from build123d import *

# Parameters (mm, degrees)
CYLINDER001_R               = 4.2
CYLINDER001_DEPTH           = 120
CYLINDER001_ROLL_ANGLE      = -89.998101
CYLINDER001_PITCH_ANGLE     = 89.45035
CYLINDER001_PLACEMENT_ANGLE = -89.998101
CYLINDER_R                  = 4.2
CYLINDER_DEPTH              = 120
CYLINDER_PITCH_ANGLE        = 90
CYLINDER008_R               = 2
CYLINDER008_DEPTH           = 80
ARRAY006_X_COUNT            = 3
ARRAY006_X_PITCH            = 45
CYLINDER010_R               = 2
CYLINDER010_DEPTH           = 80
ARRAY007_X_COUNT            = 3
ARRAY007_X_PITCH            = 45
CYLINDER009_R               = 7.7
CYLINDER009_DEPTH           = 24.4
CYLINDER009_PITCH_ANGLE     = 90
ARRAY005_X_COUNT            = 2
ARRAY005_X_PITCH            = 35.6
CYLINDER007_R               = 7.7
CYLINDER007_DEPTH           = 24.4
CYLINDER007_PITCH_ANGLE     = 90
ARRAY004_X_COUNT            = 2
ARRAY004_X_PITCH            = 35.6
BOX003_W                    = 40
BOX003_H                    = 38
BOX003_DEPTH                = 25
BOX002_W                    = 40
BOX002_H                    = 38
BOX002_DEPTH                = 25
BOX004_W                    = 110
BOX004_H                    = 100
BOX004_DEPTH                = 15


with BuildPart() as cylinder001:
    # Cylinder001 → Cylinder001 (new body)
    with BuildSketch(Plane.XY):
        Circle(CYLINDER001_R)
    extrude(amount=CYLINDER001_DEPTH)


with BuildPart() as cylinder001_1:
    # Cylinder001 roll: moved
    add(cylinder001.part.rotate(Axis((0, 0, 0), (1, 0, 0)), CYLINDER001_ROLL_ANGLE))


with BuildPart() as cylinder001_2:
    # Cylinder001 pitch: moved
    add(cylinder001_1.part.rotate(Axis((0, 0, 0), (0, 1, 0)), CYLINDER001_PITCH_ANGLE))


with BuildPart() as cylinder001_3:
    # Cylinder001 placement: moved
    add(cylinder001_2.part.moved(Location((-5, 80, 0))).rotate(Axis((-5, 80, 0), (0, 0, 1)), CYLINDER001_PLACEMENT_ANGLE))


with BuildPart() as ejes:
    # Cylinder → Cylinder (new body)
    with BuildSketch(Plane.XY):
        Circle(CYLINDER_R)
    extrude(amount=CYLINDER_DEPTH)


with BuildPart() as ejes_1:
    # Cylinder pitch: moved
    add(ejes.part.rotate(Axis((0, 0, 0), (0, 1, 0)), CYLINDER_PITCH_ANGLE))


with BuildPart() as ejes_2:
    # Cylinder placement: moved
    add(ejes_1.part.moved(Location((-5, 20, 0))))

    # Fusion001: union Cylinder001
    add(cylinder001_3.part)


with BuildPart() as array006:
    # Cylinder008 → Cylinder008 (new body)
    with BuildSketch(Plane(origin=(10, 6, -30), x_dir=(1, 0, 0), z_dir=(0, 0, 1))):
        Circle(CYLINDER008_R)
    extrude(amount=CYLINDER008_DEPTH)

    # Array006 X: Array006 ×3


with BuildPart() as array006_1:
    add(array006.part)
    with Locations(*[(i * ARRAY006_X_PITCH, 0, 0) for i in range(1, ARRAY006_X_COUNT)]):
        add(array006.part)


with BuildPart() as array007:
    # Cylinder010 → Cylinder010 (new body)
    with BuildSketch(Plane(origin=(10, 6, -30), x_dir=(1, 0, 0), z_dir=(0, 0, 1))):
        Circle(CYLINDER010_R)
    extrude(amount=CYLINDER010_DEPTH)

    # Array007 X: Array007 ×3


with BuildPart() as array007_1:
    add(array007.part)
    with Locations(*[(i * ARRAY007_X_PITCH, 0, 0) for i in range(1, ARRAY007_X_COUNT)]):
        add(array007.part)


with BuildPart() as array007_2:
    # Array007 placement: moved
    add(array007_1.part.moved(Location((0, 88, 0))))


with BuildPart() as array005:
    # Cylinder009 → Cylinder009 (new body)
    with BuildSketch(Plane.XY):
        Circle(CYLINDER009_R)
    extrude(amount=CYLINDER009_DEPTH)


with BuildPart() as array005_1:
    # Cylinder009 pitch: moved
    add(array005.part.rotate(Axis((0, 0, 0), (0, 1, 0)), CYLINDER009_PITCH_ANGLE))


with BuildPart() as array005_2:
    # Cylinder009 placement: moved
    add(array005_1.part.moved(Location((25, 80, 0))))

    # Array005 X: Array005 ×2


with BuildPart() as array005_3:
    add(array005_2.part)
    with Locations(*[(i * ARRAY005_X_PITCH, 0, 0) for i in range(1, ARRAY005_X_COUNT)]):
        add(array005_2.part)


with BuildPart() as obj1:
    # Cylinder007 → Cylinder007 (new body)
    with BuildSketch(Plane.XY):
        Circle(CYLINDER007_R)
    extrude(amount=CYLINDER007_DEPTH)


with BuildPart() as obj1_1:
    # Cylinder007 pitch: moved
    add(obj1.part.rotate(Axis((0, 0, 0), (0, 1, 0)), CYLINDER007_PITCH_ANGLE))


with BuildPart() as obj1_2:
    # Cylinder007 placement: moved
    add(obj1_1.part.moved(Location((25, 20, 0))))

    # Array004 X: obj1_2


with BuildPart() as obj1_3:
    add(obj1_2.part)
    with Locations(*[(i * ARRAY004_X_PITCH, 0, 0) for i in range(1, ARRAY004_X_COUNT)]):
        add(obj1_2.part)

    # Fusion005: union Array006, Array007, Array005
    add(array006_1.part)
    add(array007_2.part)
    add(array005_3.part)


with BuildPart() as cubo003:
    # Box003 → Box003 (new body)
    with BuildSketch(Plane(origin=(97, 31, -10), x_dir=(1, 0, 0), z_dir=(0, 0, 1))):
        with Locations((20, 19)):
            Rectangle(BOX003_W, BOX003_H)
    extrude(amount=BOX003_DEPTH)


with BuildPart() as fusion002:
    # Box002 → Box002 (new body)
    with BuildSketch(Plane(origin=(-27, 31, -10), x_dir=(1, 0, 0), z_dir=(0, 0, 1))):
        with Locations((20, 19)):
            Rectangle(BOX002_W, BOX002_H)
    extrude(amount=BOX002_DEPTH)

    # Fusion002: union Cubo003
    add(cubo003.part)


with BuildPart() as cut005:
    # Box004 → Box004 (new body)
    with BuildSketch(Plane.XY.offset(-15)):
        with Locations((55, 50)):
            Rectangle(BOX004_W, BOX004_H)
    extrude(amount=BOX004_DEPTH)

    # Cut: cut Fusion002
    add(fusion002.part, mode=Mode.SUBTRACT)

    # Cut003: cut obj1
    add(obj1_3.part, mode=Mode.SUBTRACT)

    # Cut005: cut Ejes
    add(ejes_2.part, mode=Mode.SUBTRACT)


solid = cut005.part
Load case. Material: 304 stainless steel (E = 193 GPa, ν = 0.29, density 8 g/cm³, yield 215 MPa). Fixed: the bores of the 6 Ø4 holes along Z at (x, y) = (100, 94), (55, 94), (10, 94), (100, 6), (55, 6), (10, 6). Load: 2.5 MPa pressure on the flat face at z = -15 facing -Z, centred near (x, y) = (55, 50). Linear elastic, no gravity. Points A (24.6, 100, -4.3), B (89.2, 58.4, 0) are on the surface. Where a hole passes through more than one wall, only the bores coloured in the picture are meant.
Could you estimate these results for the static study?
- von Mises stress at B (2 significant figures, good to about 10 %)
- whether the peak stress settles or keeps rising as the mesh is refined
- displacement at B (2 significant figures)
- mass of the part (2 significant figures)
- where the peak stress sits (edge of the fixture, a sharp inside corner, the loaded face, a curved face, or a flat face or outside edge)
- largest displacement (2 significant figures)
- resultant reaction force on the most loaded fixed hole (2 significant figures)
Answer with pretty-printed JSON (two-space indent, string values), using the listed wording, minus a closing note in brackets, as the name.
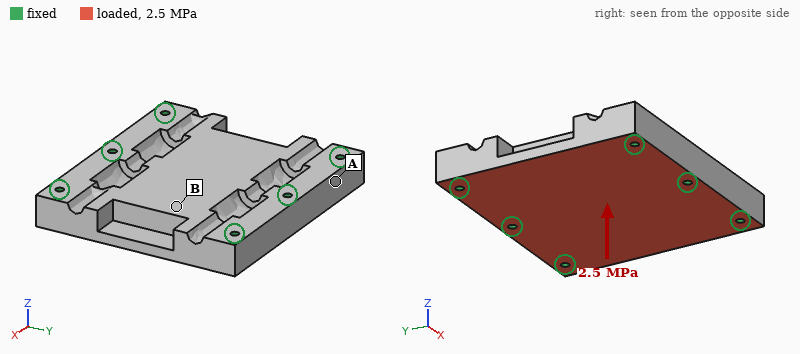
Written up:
{
  "von Mises stress at B": "34 MPa",
  "whether the peak stress settles or keeps rising as the mesh is refined": "keeps rising",
  "displacement at B": "17 µm",
  "mass of the part": "1.1 kg",
  "where the peak stress sits": "edge of the fixture",
  "largest displacement": "24 µm",
  "resultant reaction force on the most loaded fixed hole": "5.5 kN"
}
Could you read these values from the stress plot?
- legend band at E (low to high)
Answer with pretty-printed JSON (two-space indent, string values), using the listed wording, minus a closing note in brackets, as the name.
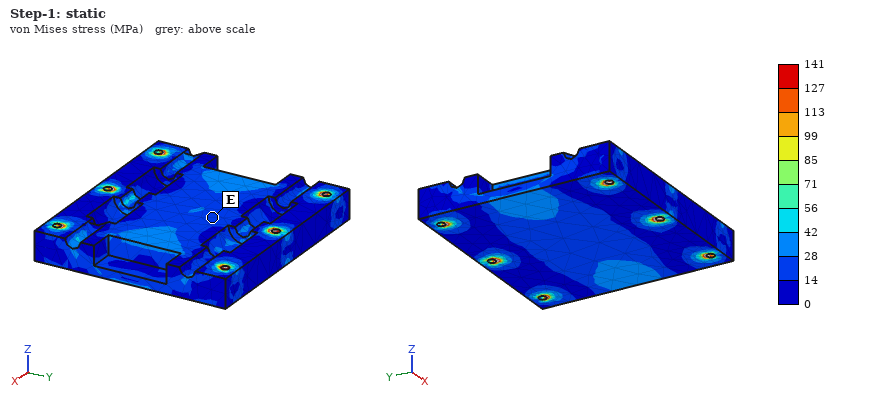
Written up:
{
  "legend band at E": "14 to 28 MPa"
}
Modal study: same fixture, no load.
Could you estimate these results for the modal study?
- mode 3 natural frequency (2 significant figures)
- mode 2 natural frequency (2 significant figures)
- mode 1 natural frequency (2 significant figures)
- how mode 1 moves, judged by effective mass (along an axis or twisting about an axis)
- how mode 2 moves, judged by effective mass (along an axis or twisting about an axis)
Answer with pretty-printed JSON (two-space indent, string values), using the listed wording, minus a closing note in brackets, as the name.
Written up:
{
  "mode 3 natural frequency": "13 kHz",
  "mode 2 natural frequency": "8200 Hz",
  "mode 1 natural frequency": "6600 Hz",
  "how mode 1 moves, judged by effective mass": "along Z",
  "how mode 2 moves, judged by effective mass": "twisting about Y"
}
